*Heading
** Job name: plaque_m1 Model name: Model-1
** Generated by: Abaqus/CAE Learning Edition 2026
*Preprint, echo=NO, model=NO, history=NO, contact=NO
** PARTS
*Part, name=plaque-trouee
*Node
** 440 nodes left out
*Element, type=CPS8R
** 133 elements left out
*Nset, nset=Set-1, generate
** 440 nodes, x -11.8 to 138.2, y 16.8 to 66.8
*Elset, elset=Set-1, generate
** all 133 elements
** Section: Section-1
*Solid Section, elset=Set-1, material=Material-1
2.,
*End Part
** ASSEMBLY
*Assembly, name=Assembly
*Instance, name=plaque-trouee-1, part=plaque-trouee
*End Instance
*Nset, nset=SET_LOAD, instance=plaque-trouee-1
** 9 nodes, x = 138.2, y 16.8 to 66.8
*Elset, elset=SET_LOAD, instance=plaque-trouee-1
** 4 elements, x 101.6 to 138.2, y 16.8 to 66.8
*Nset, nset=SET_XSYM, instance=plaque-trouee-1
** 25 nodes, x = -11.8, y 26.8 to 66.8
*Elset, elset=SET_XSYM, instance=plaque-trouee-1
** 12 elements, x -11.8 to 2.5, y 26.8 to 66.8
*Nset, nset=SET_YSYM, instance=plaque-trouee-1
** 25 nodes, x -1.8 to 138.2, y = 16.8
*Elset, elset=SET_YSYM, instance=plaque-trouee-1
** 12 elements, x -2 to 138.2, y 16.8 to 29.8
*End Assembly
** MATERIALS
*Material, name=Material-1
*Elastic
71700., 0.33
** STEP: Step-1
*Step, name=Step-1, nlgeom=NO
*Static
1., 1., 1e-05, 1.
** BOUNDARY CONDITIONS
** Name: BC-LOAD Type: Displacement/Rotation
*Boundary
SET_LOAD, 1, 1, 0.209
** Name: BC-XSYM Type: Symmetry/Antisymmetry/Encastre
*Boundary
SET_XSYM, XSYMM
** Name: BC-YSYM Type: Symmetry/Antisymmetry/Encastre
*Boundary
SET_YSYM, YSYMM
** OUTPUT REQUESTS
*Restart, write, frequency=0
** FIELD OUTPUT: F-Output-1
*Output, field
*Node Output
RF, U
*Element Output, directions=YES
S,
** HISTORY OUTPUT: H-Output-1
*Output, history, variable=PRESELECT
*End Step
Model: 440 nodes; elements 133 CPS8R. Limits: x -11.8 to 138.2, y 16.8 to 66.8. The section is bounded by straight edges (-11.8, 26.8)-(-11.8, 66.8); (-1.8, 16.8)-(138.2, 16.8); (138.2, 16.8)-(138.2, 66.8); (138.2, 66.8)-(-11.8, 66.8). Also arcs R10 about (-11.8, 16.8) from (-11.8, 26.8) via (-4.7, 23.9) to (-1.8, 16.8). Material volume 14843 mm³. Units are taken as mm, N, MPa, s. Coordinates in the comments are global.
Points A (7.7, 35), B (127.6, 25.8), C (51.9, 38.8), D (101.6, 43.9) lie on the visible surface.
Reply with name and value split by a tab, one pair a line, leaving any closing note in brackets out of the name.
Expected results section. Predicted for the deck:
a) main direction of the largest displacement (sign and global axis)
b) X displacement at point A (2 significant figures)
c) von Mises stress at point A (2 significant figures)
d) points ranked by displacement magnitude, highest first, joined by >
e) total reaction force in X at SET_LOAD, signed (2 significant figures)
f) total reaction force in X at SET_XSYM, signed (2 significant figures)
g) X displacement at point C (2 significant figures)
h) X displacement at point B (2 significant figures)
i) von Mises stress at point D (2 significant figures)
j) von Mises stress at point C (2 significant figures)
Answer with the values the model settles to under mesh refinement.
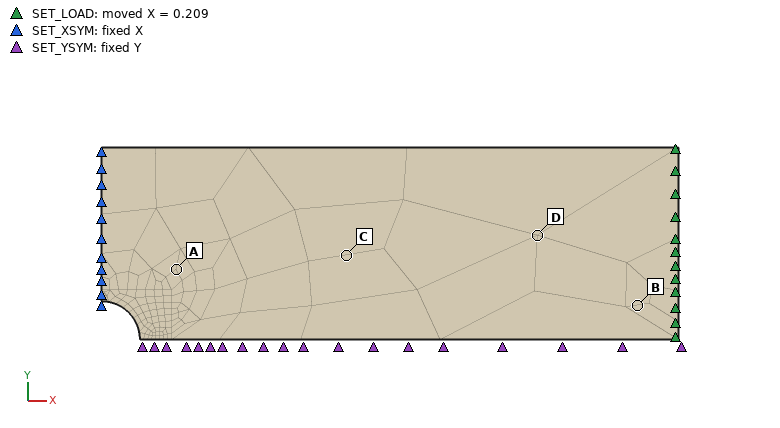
main direction of the largest displacement	+X
X displacement at point A	0.033 mm
von Mises stress at point A	120 MPa
points ranked by displacement magnitude, highest first, joined by >	B > D > C > A
total reaction force in X at SET_LOAD, signed	9700 N
total reaction force in X at SET_XSYM, signed	-9700 N
X displacement at point C	0.093 mm
X displacement at point B	0.19 mm
von Mises stress at point D	97 MPa
von Mises stress at point C	95 MPa
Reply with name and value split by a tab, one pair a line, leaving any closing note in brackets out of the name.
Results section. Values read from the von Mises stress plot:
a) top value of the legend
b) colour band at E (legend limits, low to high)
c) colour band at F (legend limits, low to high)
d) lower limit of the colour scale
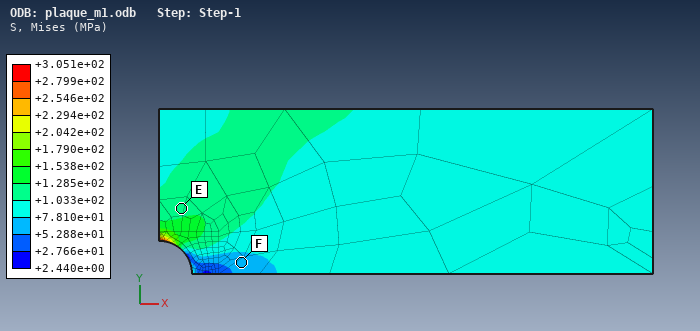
top value of the legend	+3.051e+02 MPa
colour band at E	+1.033e+02 to +1.285e+02 MPa
colour band at F	+5.288e+01 to +7.810e+01 MPa
lower limit of the colour scale	+2.440e+00 MPa
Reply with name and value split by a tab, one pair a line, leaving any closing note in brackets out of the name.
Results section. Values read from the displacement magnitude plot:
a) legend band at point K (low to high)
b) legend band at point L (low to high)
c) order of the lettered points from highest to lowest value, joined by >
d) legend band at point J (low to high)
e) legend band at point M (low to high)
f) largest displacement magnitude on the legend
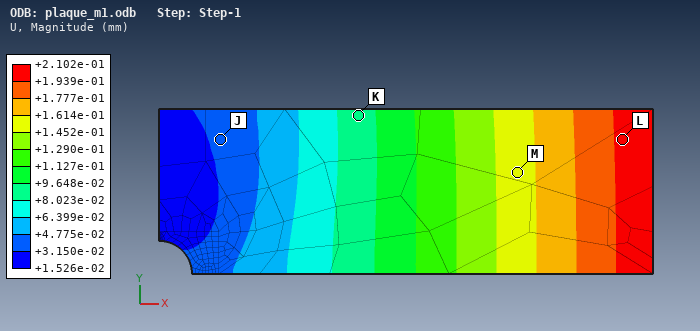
legend band at point K	+8.023e-02 to +9.648e-02 mm
legend band at point L	+1.939e-01 to +2.102e-01 mm
order of the lettered points from highest to lowest value, joined by >	L > M > K > J
legend band at point J	+3.150e-02 to +4.775e-02 mm
legend band at point M	+1.452e-01 to +1.614e-01 mm
largest displacement magnitude on the legend	+2.102e-01 mm
